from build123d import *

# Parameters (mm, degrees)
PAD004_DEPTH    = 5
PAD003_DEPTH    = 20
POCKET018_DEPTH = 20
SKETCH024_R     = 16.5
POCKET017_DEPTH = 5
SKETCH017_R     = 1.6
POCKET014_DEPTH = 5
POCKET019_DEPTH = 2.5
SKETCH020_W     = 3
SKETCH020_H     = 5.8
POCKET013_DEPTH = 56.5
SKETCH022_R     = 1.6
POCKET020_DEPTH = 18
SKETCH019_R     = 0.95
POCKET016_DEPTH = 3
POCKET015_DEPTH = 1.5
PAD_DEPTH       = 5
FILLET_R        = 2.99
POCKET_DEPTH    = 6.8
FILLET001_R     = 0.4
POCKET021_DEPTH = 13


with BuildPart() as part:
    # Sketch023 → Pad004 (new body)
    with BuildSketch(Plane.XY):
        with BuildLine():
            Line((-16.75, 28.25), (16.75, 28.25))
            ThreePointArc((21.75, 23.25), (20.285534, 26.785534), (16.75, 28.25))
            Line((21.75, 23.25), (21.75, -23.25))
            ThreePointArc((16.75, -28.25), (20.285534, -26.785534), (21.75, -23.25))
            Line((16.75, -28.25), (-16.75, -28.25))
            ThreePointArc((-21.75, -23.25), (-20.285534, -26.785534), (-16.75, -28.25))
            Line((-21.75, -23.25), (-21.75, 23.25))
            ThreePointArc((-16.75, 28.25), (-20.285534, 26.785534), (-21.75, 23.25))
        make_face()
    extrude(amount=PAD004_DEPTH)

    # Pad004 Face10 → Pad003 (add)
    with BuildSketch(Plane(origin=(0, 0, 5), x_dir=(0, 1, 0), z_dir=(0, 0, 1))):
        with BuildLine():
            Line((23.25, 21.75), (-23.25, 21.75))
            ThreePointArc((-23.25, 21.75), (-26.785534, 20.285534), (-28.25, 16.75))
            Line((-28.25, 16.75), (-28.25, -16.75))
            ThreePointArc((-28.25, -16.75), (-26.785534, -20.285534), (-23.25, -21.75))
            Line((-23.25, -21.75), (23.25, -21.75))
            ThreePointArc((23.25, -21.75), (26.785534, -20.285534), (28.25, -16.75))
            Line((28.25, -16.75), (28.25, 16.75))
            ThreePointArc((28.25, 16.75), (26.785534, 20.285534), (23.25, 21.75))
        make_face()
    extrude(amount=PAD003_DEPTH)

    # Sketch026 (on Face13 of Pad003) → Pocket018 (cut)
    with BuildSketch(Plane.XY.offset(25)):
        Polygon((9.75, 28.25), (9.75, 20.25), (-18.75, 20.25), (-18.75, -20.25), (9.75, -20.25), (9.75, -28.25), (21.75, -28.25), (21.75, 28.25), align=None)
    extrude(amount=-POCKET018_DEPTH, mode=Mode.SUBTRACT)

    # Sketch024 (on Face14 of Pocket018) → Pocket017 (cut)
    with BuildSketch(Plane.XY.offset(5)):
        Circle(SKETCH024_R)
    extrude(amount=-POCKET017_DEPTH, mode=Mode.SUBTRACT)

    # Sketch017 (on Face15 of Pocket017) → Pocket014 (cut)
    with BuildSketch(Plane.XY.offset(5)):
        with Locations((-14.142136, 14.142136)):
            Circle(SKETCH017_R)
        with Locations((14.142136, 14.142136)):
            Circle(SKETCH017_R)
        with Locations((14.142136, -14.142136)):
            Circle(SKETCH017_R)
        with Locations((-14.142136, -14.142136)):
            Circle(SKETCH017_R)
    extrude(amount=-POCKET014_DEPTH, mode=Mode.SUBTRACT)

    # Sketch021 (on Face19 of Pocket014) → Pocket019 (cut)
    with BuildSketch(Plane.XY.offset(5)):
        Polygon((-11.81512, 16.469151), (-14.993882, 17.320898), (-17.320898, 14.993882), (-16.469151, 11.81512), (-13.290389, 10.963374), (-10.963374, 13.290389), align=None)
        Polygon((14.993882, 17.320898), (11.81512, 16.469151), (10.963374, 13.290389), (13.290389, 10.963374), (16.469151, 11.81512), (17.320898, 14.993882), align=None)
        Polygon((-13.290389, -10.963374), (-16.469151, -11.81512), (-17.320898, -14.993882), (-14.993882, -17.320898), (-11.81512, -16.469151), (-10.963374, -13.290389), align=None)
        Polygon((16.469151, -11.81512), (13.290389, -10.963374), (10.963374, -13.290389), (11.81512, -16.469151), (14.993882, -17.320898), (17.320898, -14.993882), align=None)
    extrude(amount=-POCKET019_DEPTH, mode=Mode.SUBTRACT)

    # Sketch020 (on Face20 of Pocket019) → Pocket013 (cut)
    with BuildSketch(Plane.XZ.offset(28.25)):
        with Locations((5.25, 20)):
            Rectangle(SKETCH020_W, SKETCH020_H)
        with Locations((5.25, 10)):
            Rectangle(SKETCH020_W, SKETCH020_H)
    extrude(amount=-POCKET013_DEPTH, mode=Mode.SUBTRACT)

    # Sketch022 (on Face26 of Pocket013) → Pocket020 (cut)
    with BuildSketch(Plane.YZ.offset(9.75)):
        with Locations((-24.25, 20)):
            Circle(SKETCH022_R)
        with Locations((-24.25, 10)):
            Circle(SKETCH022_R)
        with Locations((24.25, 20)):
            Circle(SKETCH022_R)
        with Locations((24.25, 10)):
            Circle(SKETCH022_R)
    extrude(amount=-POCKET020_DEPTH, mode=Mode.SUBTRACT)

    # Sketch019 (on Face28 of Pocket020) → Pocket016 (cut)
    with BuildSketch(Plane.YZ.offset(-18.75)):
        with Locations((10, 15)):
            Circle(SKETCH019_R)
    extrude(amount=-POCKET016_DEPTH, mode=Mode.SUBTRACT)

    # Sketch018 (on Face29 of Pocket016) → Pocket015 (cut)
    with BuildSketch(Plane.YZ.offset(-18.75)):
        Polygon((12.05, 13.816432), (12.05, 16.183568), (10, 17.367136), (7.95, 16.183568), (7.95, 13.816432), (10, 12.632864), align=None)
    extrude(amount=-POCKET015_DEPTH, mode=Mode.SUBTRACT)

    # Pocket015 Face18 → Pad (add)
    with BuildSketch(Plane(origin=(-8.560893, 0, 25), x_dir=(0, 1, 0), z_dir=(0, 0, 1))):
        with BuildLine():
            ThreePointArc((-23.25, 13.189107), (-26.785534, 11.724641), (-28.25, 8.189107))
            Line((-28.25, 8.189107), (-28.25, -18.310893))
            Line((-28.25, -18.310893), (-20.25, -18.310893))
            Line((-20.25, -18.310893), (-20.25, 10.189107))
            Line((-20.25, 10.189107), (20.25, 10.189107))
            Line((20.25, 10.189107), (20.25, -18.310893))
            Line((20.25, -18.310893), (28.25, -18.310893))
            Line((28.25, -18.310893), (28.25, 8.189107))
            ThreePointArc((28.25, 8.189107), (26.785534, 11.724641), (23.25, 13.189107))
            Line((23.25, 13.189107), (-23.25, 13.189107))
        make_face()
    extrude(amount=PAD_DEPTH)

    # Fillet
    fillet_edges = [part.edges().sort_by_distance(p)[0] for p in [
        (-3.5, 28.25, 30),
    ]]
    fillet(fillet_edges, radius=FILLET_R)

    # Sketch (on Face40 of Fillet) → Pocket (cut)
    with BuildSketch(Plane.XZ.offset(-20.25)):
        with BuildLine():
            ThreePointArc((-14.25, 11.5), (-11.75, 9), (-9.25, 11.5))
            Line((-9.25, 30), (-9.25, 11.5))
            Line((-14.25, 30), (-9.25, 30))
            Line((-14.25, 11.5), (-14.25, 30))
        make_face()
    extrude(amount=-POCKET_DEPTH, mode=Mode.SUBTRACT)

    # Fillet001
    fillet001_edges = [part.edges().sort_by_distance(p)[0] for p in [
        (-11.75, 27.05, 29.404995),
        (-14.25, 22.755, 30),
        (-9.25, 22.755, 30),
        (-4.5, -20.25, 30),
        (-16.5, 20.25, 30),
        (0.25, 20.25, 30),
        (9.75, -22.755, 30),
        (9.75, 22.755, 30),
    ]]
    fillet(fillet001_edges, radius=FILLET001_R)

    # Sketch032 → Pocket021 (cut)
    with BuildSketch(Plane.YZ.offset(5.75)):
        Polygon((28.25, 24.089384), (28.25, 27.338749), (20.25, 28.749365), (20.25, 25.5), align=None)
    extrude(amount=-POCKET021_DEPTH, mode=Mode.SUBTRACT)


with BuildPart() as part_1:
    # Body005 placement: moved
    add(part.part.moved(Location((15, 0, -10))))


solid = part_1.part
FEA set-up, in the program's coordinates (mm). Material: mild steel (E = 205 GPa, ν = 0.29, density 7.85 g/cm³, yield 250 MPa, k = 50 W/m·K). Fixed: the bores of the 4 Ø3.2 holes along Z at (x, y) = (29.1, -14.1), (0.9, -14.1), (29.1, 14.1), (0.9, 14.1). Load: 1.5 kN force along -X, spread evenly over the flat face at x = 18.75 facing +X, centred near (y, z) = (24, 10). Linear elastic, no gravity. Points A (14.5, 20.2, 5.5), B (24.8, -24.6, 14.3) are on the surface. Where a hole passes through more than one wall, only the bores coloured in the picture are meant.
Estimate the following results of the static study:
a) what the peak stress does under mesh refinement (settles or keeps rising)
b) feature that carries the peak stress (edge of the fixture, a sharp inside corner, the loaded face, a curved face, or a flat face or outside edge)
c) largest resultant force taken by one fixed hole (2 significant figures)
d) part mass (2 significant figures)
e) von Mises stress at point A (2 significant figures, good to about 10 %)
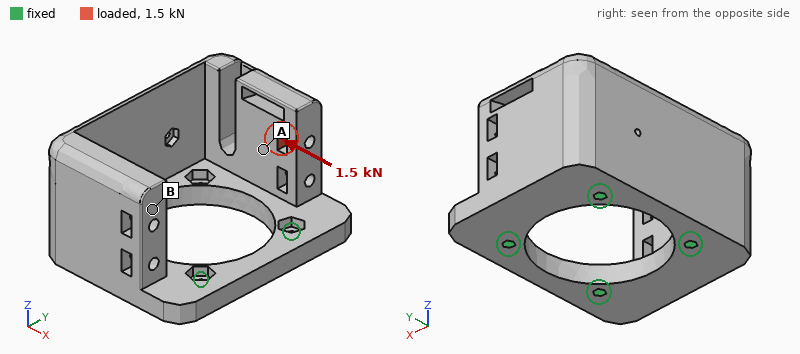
keeps rising
edge of the fixture
1.4 kN
160 g
33 MPa
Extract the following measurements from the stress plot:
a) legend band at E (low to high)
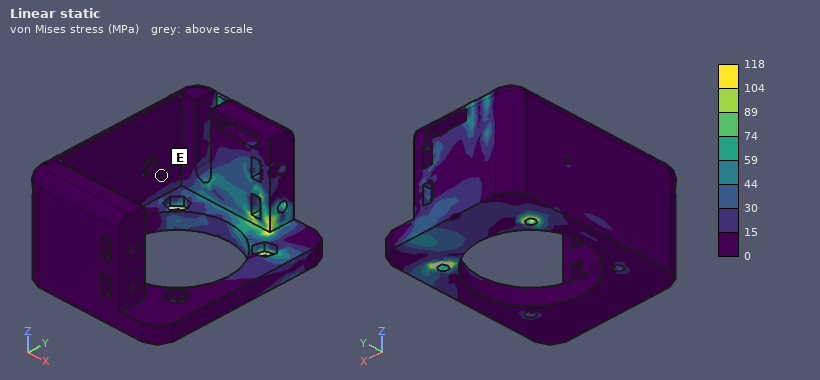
0 to 15 MPa
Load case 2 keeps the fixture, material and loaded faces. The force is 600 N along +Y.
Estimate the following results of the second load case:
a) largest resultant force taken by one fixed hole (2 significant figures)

490 N
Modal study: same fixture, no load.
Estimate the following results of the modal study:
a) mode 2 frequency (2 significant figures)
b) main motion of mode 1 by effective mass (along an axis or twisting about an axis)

5100 Hz
along Y
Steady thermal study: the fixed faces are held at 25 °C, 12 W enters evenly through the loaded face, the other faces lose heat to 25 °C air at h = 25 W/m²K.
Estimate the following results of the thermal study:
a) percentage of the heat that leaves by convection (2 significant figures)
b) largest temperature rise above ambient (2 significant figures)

24 %
56 K
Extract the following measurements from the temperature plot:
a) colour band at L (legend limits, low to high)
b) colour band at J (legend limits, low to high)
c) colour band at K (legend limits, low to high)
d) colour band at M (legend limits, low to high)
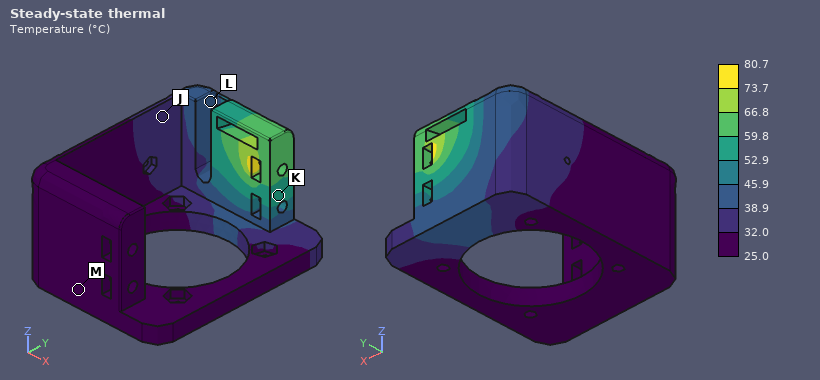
38.9 to 45.9 °C
32.0 to 38.9 °C
52.9 to 59.8 °C
25.0 to 32.0 °C
